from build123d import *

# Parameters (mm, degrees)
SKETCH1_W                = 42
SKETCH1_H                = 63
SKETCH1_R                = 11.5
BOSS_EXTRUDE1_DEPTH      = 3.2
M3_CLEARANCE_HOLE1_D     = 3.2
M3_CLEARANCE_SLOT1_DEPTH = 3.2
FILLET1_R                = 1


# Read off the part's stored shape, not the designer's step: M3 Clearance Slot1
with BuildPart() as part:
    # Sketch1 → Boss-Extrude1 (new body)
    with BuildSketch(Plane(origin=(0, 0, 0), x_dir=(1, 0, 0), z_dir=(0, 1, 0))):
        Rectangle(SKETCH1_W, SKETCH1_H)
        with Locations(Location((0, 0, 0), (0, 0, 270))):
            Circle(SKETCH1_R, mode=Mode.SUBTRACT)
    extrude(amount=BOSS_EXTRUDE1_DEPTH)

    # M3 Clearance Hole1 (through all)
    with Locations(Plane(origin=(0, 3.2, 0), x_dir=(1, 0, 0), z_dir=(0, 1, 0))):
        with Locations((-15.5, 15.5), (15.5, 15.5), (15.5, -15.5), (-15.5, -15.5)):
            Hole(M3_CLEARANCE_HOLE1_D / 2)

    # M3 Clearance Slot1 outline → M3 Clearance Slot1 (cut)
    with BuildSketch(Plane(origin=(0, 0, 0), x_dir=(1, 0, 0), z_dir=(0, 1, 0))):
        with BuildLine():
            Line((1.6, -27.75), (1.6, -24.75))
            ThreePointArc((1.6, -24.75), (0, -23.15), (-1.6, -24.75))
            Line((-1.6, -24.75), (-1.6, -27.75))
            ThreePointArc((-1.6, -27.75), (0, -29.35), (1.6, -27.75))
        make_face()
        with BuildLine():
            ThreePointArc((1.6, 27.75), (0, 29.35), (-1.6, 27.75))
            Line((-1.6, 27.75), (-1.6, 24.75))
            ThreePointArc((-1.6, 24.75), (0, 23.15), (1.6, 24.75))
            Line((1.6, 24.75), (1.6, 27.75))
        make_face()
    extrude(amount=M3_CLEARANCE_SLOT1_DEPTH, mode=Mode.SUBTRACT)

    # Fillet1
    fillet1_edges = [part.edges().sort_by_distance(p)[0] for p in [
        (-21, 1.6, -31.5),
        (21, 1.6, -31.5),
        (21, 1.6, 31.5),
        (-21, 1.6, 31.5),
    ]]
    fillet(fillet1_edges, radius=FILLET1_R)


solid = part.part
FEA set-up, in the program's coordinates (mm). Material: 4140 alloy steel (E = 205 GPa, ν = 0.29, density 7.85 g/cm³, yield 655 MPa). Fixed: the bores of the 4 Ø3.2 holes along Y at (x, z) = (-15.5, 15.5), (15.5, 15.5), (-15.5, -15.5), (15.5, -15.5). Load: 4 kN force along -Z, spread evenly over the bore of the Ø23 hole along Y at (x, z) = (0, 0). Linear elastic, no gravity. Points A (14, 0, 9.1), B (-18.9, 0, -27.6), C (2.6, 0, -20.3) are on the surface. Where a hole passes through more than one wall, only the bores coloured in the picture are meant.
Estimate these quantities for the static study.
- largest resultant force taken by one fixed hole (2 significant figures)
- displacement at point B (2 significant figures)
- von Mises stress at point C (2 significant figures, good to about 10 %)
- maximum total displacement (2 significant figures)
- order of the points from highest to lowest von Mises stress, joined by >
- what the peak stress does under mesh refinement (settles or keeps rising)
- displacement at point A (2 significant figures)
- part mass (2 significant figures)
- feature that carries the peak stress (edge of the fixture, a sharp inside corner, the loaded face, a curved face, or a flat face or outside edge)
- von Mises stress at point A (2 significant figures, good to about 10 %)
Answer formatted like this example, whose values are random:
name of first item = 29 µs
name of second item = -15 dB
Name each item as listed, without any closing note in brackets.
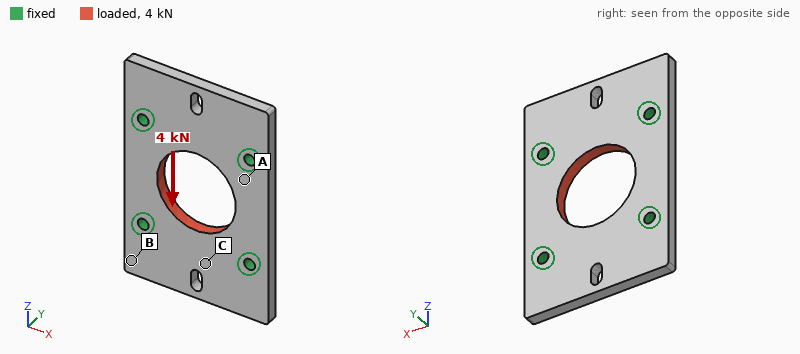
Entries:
largest resultant force taken by one fixed hole = 1.0 kN
displacement at point B = 0.64 µm
von Mises stress at point C = 14 MPa
maximum total displacement = 2.5 µm
order of the points from highest to lowest von Mises stress, joined by > = A > C > B
what the peak stress does under mesh refinement = keeps rising
displacement at point A = 0.76 µm
part mass = 54 g
feature that carries the peak stress = edge of the fixture
von Mises stress at point A = 23 MPa
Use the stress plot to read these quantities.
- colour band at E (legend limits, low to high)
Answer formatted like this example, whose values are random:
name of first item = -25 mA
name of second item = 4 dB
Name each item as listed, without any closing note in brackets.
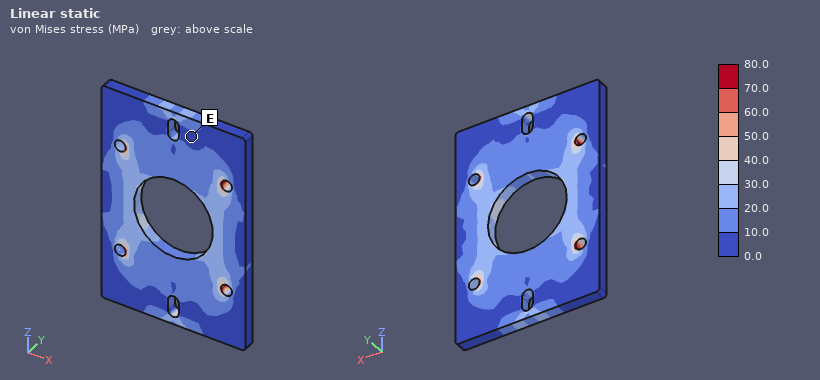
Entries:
colour band at E = 0.0 to 10.0 MPa
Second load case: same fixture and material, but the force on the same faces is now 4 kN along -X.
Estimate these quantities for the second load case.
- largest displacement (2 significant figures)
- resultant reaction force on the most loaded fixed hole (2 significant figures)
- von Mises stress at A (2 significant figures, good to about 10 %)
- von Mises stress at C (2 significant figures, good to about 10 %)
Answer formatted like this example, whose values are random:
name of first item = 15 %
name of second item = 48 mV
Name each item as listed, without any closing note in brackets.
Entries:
largest displacement = 3.8 µm
resultant reaction force on the most loaded fixed hole = 1.0 kN
von Mises stress at A = 26 MPa
von Mises stress at C = 8.7 MPa
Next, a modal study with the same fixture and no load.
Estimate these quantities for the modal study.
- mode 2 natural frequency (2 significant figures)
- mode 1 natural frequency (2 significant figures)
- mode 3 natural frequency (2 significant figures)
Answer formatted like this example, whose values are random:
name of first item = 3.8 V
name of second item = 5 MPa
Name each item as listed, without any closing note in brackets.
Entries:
mode 2 natural frequency = 8400 Hz
mode 1 natural frequency = 8300 Hz
mode 3 natural frequency = 13 kHz
